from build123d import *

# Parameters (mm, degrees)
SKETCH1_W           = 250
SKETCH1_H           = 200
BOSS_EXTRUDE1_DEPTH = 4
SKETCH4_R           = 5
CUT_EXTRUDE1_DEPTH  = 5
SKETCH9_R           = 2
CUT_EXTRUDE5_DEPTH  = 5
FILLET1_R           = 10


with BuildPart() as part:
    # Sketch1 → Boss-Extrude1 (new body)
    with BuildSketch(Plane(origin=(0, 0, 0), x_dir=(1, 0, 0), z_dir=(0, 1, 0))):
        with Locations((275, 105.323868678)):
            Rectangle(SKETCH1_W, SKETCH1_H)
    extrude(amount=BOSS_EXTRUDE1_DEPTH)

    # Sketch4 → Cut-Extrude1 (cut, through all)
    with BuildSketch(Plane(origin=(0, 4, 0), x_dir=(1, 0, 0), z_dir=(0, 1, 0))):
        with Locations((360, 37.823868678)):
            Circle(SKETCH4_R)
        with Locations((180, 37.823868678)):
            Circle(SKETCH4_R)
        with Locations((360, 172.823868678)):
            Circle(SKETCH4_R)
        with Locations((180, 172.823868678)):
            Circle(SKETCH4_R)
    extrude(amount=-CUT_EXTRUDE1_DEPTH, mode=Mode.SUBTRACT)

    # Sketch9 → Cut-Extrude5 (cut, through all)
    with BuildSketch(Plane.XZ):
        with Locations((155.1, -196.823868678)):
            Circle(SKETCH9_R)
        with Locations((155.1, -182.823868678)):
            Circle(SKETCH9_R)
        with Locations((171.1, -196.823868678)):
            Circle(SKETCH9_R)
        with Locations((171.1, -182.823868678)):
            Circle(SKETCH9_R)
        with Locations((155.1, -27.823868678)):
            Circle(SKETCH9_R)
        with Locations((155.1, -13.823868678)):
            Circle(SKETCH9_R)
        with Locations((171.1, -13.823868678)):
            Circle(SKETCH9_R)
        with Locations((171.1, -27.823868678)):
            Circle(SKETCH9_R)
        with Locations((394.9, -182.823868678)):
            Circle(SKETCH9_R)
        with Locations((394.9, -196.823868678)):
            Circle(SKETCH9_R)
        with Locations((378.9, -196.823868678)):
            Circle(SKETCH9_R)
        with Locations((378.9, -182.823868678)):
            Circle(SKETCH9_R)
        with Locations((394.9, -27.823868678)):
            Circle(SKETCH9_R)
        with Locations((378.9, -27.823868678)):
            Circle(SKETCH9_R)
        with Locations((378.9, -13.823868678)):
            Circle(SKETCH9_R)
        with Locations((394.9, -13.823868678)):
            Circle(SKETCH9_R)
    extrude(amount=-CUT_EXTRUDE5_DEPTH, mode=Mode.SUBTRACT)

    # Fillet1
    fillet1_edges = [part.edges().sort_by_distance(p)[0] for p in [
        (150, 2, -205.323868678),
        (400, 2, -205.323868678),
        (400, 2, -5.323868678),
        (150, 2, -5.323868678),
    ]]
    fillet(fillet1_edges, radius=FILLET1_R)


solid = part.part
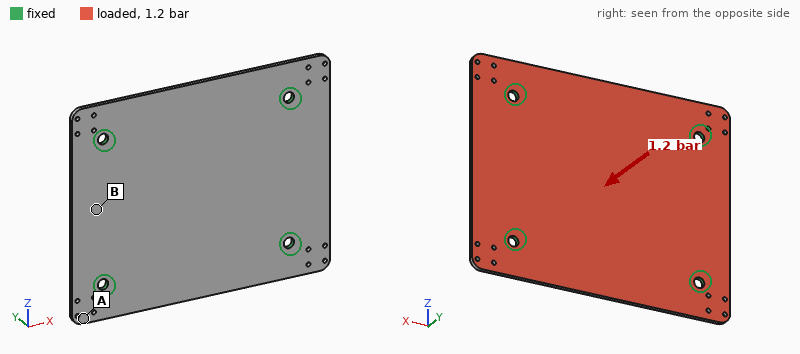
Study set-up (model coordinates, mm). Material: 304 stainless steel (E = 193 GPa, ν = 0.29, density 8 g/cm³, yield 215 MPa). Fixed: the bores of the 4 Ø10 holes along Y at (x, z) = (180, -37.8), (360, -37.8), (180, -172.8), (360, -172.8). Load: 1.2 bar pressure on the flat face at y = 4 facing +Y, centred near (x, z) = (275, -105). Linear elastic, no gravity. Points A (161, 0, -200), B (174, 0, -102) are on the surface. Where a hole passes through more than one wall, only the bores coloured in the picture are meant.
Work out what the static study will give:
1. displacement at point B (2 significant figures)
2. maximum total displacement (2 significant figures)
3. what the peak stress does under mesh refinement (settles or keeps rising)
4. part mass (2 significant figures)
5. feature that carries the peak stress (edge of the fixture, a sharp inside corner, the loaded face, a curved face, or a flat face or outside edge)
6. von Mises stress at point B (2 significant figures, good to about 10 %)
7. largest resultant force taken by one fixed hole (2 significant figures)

0.12 mm
0.46 mm
keeps rising
1.6 kg
edge of the fixture
44 MPa
1.5 kN
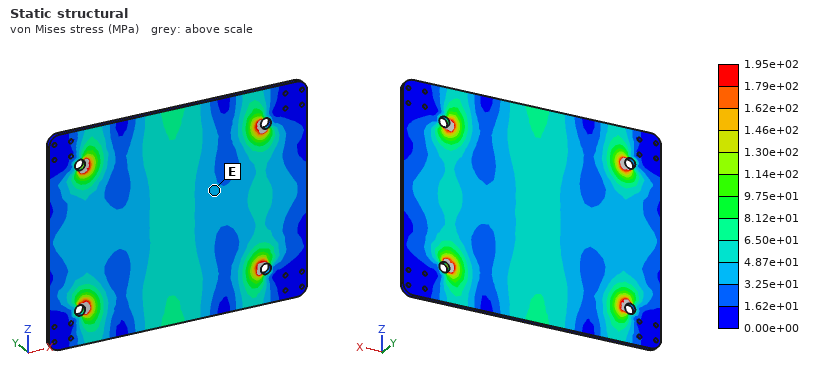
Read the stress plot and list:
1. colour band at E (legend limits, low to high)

3.25e+01 to 4.87e+01 MPa
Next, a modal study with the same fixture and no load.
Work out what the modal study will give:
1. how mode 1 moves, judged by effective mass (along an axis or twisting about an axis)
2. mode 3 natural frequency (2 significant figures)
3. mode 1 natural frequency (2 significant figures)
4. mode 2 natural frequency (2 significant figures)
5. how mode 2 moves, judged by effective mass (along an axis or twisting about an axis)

along Y
900 Hz
540 Hz
710 Hz
twisting about X
